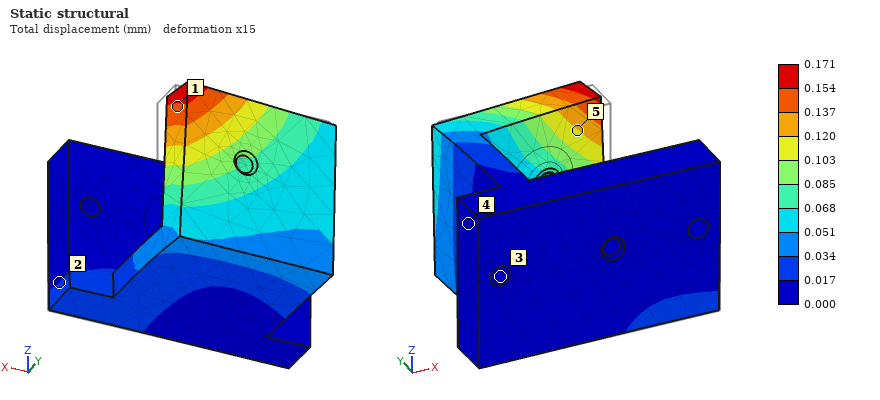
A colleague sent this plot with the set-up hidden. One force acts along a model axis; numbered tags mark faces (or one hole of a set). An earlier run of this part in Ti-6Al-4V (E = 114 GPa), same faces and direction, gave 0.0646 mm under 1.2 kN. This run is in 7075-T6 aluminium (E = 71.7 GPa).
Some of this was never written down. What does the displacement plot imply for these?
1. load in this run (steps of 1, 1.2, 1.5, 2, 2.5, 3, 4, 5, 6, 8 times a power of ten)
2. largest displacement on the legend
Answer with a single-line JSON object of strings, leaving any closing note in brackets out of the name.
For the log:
{"load in this run": "2 kN", "largest displacement on the legend": "0.171 mm"}
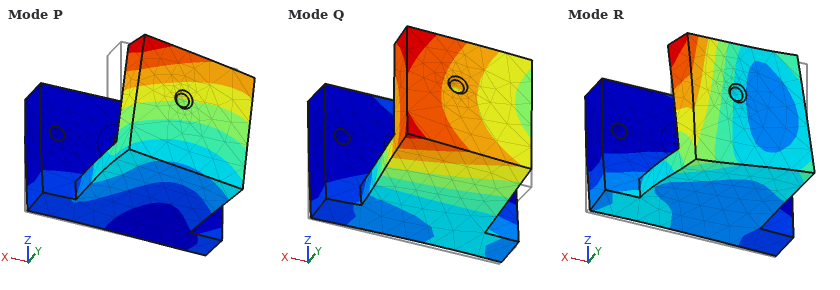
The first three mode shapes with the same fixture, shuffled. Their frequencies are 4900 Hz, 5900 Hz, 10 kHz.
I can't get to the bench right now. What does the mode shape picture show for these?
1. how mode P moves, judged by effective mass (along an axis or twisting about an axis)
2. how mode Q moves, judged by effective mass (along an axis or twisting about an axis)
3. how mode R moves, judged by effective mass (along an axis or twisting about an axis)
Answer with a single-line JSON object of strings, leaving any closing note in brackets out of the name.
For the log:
{"how mode P moves, judged by effective mass": "along X", "how mode Q moves, judged by effective mass": "along Z", "how mode R moves, judged by effective mass": "along Y"}
